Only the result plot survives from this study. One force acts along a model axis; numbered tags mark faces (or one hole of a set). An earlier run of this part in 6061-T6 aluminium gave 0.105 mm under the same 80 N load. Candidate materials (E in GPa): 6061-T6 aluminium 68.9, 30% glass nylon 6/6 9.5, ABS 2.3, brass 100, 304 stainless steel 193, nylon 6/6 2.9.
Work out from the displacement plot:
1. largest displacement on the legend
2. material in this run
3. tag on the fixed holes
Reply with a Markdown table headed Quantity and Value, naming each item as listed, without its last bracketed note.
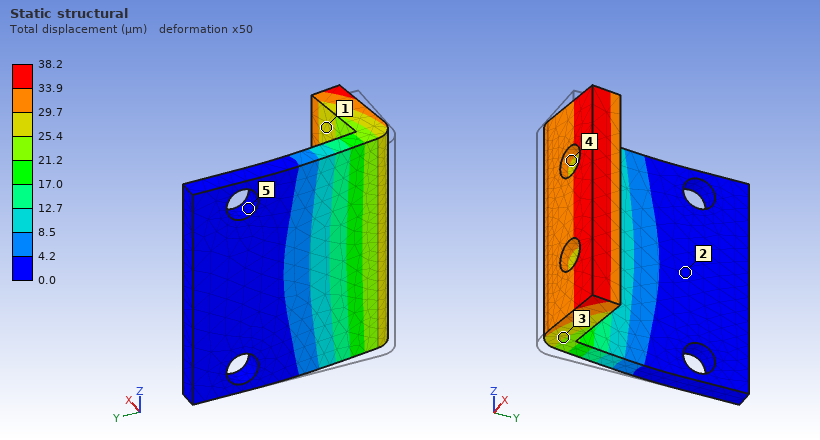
| Quantity | Value |
|---|---|
| largest displacement on the legend | 38.2 µm |
| material in this run | 304 stainless steel |
| tag on the fixed holes | 5 |
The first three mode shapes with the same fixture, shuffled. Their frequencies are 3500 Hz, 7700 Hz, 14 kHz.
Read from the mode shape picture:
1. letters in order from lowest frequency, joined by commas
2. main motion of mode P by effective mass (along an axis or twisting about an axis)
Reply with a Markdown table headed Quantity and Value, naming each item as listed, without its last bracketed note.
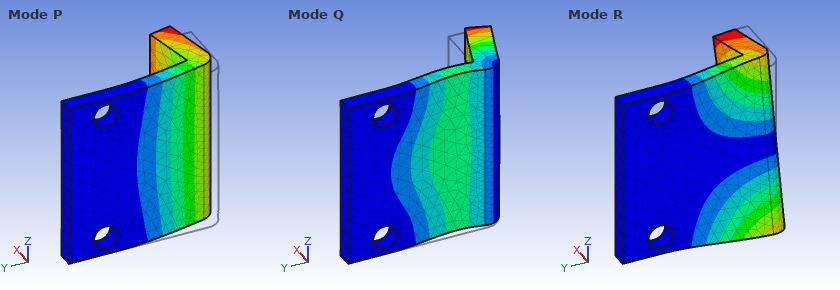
| Quantity | Value |
|---|---|
| letters in order from lowest frequency, joined by commas | P, R, Q |
| main motion of mode P by effective mass | along X |
